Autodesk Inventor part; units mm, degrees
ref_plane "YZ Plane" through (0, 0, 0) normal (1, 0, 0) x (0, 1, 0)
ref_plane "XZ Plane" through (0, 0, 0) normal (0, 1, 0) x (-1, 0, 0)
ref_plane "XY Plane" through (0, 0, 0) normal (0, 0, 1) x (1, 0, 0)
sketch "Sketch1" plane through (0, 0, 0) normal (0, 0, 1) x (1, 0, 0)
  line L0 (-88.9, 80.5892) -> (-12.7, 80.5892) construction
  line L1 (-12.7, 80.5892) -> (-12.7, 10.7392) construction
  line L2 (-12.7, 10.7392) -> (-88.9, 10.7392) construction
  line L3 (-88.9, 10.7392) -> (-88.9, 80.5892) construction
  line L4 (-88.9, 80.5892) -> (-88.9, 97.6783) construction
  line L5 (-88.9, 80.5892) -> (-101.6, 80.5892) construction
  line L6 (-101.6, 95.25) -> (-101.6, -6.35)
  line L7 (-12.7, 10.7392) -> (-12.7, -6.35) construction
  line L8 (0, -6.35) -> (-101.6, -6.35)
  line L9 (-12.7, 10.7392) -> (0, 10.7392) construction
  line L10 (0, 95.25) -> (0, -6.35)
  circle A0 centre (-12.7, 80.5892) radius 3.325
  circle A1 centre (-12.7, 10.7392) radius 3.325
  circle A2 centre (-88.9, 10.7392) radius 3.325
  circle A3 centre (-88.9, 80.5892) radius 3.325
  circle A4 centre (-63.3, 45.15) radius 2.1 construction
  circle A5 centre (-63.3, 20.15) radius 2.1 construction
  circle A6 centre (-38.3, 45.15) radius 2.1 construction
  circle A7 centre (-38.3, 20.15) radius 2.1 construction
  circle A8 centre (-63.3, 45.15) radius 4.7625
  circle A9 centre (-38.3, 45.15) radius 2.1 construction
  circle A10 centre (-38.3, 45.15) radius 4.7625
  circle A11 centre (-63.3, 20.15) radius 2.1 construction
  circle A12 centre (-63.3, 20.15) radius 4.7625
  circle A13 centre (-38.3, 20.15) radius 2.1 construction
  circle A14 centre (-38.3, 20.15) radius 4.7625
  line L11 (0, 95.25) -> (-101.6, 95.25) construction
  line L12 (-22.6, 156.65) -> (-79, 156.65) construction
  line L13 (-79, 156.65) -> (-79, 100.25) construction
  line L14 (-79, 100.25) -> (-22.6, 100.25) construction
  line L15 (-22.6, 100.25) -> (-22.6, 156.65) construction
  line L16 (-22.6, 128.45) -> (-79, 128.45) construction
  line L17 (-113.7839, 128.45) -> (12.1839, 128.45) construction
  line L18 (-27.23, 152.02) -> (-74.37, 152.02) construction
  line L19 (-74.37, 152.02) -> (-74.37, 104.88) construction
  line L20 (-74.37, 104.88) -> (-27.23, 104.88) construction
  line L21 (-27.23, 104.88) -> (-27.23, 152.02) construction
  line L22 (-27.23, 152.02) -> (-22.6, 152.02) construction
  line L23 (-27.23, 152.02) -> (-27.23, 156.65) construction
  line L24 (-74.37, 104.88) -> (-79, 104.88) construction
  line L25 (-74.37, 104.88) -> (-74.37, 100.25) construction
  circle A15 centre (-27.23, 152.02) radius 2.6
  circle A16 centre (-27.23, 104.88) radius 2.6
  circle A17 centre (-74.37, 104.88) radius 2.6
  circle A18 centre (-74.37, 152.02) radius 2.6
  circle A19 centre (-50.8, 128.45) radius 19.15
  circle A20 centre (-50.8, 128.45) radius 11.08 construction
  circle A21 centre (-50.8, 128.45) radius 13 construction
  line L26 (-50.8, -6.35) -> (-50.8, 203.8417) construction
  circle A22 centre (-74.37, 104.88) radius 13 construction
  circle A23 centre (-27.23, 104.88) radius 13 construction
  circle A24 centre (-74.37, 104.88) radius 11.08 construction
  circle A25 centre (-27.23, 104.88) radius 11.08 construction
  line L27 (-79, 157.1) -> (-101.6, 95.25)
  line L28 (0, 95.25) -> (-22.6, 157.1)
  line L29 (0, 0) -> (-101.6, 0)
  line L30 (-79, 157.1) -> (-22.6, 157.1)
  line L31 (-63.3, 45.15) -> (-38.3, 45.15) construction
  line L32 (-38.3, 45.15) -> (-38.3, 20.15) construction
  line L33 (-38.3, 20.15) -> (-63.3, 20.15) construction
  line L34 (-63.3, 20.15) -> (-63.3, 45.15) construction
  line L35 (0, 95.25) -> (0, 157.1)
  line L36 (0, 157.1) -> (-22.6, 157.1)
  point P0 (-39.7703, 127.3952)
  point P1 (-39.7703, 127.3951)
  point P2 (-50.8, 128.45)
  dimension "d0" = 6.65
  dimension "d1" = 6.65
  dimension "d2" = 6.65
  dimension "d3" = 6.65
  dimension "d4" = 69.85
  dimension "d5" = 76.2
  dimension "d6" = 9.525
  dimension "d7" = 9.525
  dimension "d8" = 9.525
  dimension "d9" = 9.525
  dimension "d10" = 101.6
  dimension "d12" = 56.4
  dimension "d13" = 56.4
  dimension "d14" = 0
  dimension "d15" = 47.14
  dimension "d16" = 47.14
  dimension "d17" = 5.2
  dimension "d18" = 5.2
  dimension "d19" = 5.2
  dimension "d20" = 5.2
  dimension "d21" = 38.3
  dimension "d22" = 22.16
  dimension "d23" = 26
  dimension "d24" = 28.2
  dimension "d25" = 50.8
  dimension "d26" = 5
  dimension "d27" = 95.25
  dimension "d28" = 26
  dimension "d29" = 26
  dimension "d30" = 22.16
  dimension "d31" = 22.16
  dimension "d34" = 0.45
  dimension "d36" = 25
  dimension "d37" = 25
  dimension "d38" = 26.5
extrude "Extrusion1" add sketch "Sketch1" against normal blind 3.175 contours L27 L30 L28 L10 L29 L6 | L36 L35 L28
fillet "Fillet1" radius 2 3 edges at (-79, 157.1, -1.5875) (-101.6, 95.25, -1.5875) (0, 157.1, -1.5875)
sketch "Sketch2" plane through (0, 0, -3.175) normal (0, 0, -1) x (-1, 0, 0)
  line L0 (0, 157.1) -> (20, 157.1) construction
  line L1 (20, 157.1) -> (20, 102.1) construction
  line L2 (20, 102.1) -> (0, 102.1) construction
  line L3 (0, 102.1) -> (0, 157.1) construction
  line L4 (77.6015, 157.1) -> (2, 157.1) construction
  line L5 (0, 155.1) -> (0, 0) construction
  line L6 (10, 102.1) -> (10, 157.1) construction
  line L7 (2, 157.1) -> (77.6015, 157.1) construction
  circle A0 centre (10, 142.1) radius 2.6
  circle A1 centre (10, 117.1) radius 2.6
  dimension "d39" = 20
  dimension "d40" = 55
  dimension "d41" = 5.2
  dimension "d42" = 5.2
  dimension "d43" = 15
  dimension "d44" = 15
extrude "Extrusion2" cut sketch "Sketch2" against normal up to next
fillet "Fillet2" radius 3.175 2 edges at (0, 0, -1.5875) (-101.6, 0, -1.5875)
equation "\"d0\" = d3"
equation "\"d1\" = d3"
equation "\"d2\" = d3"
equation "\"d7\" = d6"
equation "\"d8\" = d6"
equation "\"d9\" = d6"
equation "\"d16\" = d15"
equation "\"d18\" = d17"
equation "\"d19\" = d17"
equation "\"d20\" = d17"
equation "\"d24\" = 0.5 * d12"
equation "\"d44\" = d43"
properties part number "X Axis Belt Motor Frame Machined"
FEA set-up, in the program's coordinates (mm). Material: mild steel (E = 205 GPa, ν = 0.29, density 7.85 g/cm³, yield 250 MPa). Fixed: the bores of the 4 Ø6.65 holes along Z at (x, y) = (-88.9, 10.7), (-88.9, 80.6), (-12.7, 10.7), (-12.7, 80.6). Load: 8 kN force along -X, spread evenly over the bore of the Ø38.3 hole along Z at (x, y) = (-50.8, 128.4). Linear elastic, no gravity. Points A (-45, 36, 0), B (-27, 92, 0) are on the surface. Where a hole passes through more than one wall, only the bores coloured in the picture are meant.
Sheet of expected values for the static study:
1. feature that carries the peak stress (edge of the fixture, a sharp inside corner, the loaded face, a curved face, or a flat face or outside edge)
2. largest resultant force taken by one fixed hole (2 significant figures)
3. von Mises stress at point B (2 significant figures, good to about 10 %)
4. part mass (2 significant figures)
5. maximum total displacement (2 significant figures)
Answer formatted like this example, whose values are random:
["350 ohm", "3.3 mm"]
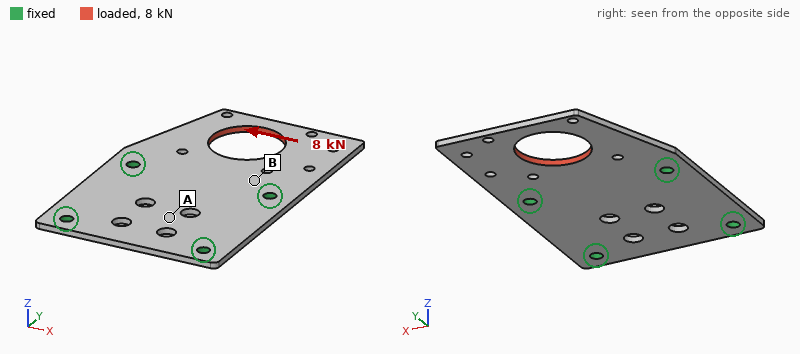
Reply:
["edge of the fixture", "6.0 kN", "54 MPa", "340 g", "68 µm"]
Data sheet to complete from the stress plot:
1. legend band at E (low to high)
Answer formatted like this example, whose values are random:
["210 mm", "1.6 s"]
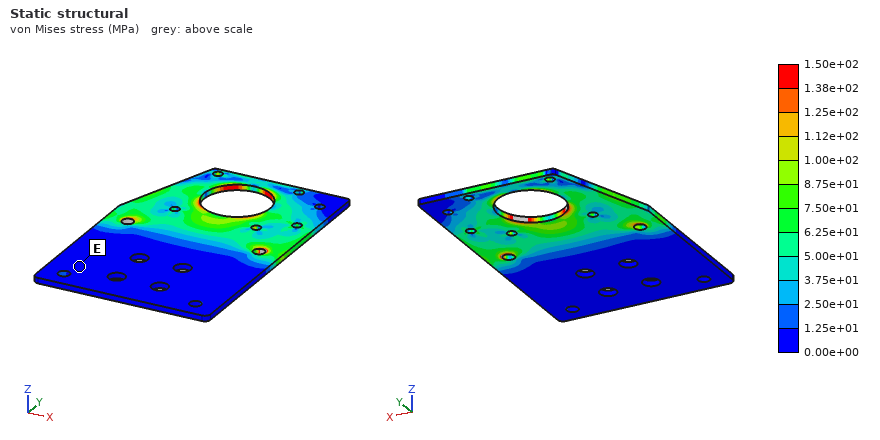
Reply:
["0.00e+00 to 1.25e+01 MPa"]
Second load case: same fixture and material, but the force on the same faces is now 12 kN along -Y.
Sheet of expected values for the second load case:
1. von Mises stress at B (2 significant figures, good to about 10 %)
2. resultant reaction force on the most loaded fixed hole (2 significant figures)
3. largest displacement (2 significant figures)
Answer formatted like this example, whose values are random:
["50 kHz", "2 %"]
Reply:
["43 MPa", "5.1 kN", "37 µm"]
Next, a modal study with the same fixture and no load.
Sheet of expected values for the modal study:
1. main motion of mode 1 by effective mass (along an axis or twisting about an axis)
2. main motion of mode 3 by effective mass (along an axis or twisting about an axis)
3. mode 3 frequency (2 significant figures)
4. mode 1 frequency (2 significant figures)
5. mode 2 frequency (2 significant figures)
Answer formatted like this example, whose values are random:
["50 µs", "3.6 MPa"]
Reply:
["along Z", "along Z", "2300 Hz", "490 Hz", "1000 Hz"]
